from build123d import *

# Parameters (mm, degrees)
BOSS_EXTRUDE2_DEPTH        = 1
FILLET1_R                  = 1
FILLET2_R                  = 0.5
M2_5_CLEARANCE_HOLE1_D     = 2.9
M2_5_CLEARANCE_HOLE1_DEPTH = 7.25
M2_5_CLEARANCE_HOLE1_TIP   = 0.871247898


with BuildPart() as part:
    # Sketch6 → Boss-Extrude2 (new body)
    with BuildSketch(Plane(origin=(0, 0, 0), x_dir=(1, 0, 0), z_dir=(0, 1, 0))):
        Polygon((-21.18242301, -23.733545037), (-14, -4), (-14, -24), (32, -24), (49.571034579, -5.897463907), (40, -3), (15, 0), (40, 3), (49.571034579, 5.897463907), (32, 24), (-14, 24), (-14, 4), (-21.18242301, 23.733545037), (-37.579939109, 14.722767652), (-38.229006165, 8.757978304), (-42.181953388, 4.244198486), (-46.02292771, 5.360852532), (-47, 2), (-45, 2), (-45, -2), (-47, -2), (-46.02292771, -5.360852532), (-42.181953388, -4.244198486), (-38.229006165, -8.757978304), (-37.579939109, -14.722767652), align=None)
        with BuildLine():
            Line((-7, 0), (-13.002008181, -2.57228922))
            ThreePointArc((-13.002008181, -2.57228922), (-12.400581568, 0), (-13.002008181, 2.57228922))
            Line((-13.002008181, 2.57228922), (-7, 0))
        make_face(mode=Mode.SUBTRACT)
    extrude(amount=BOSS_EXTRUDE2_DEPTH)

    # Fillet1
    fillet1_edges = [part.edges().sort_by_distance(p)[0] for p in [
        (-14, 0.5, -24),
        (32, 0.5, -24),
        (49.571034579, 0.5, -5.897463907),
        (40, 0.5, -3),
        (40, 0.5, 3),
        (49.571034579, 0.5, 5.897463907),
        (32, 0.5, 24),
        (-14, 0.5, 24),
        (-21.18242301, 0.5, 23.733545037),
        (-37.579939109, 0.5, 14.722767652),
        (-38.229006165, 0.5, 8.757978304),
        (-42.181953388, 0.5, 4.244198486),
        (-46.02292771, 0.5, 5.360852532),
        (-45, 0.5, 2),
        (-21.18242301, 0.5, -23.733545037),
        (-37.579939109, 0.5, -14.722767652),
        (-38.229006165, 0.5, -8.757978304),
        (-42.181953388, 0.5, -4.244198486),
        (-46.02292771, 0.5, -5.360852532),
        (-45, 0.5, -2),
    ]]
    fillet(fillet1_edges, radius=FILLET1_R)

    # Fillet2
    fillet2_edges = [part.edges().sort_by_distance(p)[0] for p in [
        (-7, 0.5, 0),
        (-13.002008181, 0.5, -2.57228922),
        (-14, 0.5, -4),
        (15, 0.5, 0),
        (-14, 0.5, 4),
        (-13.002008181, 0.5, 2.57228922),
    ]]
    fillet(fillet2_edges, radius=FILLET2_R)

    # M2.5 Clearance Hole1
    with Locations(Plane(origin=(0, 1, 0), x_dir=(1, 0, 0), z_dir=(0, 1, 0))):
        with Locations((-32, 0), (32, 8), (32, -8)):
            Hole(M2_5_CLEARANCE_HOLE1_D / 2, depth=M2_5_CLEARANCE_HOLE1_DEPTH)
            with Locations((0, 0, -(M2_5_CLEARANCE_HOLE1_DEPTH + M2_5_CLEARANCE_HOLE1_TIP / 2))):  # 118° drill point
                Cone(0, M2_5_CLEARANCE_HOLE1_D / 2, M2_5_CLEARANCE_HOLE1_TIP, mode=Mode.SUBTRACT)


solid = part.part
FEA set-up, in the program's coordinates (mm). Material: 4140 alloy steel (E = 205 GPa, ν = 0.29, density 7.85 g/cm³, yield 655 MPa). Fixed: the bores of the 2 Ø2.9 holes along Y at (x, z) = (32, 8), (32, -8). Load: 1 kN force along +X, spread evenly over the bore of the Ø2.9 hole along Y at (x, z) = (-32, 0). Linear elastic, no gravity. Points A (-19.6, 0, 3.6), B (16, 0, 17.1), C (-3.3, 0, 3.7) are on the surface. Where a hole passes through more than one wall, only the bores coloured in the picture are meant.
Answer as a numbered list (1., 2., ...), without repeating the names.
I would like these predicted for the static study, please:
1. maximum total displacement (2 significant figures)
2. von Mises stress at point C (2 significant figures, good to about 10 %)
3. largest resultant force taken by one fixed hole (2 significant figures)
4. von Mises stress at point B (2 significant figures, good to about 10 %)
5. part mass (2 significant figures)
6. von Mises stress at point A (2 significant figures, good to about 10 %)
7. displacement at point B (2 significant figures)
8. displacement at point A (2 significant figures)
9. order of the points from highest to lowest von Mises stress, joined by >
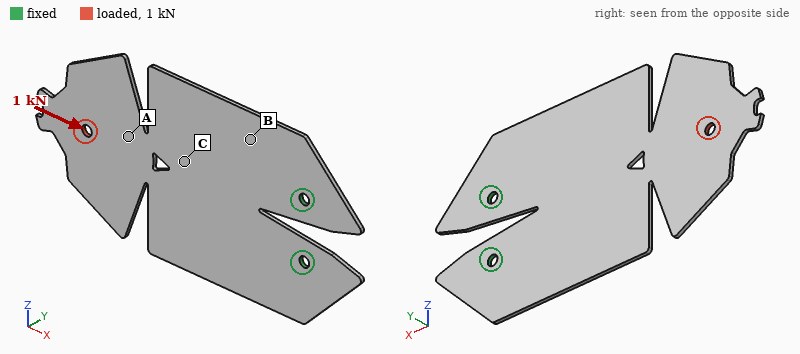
1. 17 µm
2. 45 MPa
3. 500 N
4. 16 MPa
5. 27 g
6. 67 MPa
7. 3.3 µm
8. 11 µm
9. A > C > B
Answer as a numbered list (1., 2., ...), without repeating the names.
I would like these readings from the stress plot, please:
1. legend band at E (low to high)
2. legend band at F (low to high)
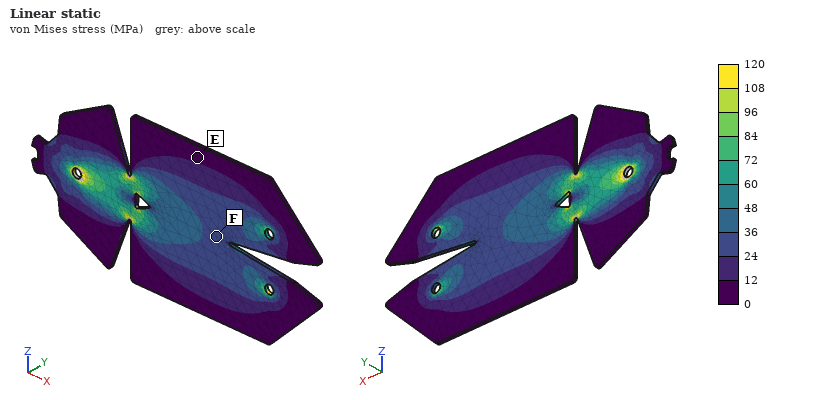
1. 0 to 12 MPa
2. 24 to 36 MPa
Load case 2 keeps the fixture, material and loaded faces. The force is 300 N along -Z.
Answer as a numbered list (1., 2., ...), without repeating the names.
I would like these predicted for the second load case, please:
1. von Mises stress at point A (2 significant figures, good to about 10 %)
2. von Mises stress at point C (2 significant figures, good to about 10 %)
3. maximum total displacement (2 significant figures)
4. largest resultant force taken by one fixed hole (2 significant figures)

1. 71 MPa
2. 31 MPa
3. 0.13 mm
4. 940 N
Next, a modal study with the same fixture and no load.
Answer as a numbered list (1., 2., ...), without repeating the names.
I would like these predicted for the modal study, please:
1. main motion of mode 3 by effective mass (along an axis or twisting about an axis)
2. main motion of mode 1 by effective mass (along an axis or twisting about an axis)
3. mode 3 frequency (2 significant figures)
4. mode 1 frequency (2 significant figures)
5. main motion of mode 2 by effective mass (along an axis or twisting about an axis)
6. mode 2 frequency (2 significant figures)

1. along Y
2. along Y
3. 770 Hz
4. 170 Hz
5. twisting about X
6. 570 Hz
